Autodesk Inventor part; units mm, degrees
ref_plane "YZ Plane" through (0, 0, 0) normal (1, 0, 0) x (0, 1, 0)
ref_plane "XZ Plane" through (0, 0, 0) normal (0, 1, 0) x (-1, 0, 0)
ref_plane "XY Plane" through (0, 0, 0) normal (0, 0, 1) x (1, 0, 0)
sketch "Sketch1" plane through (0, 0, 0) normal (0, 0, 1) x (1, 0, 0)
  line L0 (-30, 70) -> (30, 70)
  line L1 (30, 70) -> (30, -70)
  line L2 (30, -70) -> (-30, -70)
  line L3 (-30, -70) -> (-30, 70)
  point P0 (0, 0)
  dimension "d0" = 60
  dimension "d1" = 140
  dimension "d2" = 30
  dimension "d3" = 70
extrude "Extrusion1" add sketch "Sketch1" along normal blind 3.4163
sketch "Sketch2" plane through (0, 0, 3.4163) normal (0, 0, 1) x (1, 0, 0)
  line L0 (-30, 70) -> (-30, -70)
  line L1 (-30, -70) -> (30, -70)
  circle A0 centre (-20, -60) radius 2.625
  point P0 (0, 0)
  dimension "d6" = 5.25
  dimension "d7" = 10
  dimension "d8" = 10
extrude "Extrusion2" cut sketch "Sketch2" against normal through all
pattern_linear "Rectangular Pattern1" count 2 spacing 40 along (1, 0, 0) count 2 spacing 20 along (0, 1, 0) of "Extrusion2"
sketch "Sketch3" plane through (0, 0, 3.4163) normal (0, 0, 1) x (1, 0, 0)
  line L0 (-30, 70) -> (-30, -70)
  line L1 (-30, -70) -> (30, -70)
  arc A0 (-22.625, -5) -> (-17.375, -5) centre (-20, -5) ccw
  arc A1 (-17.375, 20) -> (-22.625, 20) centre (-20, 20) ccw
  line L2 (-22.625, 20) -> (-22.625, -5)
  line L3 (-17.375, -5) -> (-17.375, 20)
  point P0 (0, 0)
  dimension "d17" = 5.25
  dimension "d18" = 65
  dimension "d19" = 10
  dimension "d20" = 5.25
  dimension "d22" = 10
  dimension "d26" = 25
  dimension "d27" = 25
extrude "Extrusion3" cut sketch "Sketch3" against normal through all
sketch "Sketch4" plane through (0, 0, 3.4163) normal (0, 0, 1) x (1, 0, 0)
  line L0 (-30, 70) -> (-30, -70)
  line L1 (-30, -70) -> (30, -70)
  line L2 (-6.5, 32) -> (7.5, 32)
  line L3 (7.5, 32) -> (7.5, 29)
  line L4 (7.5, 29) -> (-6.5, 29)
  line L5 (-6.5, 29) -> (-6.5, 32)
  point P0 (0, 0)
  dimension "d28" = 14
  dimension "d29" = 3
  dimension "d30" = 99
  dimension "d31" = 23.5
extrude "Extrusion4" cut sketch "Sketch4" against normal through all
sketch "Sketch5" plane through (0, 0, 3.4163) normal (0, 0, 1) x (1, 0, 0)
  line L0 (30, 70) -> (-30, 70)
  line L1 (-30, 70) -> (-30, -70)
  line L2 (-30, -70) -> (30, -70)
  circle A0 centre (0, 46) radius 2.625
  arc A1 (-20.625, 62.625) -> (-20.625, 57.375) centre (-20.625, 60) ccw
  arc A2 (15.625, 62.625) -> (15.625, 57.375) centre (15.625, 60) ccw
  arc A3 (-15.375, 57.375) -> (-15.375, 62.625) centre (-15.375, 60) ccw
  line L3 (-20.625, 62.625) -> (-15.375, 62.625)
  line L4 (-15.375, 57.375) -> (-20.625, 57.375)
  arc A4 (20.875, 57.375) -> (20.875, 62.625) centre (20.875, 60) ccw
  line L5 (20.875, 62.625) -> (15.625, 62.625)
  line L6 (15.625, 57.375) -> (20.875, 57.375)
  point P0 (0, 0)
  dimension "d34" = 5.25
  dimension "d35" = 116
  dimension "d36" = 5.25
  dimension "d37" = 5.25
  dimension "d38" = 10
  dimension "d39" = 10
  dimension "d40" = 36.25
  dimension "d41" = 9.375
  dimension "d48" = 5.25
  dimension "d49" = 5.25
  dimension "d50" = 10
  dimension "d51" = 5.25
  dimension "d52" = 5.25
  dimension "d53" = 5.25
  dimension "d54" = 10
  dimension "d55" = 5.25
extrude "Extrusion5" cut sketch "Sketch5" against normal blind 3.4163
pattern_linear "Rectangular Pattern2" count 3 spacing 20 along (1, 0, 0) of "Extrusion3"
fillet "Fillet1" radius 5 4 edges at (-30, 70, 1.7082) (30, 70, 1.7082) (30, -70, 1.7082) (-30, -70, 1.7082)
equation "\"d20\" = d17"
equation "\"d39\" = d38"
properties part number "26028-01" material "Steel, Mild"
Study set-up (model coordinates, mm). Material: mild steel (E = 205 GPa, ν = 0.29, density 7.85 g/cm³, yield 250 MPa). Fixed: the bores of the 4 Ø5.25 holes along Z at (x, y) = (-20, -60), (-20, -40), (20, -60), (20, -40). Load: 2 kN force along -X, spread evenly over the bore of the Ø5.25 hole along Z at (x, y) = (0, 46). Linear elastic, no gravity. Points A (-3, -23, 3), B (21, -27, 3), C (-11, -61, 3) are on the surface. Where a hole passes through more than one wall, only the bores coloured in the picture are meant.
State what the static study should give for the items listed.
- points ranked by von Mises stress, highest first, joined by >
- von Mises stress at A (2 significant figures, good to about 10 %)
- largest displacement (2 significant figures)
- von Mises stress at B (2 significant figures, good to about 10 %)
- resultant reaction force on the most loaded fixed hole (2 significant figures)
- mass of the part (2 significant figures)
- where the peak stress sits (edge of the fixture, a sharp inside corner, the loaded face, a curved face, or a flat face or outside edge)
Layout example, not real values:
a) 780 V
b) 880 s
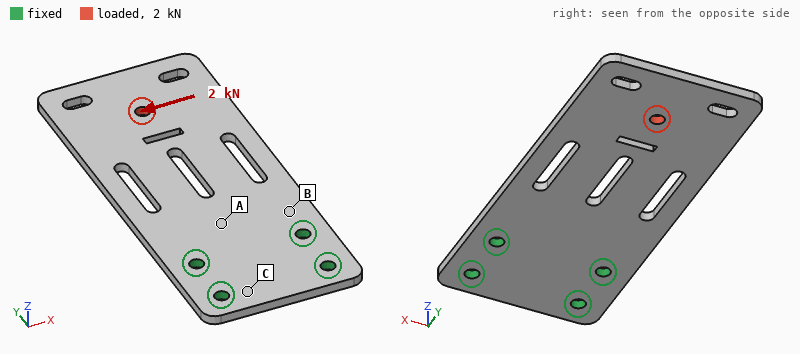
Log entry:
a) B > A > C
b) 30 MPa
c) 92 µm
d) 56 MPa
e) 3.6 kN
f) 210 g
g) a curved face
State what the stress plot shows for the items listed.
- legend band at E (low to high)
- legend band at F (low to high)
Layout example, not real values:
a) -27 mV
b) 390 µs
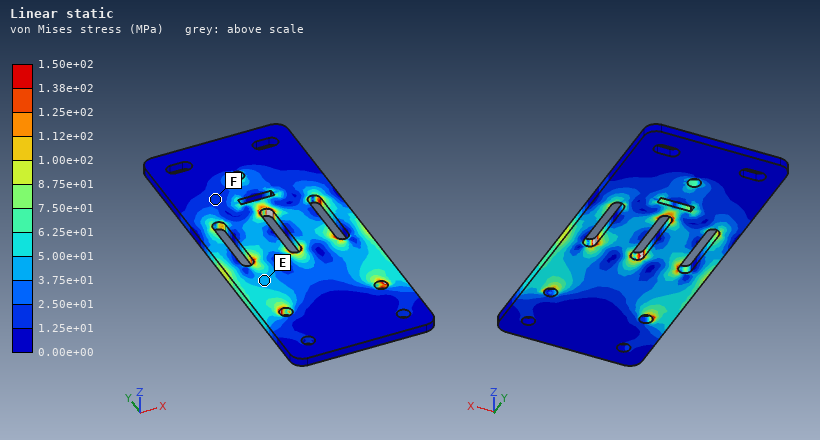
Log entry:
a) 3.75e+01 to 5.00e+01 MPa
b) 1.25e+01 to 2.50e+01 MPa
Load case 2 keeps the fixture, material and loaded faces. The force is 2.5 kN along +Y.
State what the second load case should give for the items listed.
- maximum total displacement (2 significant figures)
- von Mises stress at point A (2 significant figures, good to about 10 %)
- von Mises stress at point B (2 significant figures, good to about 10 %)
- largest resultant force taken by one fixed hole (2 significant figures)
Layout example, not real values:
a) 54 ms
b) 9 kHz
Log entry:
a) 9.3 µm
b) 9.8 MPa
c) 15 MPa
d) 1000 N
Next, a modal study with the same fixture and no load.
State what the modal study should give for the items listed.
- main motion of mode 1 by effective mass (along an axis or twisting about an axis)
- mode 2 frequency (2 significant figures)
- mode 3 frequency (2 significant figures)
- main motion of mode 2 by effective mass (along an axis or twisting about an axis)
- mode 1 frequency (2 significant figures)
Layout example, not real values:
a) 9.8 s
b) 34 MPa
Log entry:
a) along Z
b) 900 Hz
c) 1500 Hz
d) twisting about Y
e) 240 Hz
